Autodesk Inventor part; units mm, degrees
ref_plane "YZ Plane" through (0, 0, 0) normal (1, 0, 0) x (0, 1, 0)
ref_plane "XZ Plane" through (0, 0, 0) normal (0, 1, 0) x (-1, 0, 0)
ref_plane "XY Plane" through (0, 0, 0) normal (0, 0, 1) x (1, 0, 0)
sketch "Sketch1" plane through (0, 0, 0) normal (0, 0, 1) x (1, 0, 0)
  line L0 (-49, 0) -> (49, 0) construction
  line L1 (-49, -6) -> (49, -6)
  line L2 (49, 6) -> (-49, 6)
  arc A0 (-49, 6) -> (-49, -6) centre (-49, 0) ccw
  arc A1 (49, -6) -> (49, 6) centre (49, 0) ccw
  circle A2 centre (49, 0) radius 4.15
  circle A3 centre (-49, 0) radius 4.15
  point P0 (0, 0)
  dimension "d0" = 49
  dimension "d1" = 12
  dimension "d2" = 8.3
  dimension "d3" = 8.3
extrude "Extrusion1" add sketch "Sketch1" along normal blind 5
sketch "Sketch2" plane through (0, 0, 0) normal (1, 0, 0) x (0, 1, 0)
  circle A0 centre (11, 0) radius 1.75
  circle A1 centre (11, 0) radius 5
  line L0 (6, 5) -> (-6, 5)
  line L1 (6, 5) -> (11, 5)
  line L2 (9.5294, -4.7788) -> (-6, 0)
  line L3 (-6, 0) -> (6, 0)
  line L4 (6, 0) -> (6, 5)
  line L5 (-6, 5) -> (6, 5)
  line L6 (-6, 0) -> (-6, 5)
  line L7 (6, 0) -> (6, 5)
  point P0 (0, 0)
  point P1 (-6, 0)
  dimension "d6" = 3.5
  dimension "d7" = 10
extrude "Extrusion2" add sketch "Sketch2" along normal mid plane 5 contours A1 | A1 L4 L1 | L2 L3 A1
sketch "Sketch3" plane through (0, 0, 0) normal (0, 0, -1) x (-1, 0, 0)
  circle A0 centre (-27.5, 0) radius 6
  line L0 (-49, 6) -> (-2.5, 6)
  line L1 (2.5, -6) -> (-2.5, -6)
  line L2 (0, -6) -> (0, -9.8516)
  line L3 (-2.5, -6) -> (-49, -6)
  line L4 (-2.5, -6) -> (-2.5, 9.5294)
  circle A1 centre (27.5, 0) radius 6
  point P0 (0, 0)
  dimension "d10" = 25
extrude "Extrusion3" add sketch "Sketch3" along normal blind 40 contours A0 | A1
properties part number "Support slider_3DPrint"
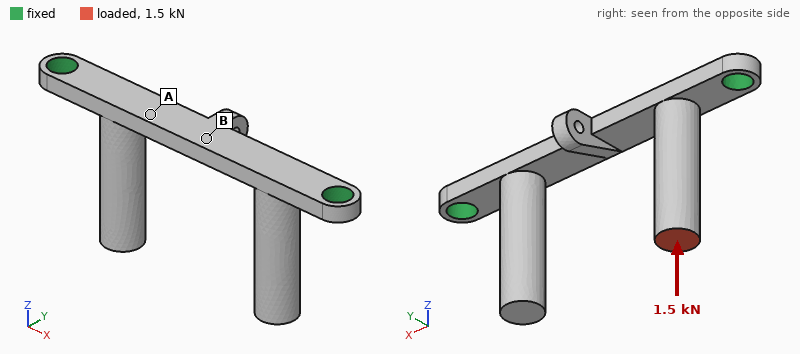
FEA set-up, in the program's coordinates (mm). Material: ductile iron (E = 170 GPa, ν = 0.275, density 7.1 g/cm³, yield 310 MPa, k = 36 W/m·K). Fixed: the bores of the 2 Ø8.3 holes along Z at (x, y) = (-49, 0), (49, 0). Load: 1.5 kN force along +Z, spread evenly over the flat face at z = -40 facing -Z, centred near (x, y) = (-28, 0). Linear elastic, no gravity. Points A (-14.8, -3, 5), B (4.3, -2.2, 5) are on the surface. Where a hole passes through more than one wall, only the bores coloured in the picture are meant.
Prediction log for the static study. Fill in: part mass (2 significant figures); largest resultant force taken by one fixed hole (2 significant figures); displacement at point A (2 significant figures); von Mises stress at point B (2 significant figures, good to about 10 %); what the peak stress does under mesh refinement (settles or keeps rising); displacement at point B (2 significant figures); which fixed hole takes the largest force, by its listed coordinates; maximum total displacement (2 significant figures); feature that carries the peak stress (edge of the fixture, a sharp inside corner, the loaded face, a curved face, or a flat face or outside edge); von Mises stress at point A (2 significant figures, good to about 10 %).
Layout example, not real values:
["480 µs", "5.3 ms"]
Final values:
["110 g", "1.3 kN", "0.11 mm", "42 MPa", "keeps rising", "0.093 mm", "(-49, 0)", "0.21 mm", "edge of the fixture", "110 MPa"]
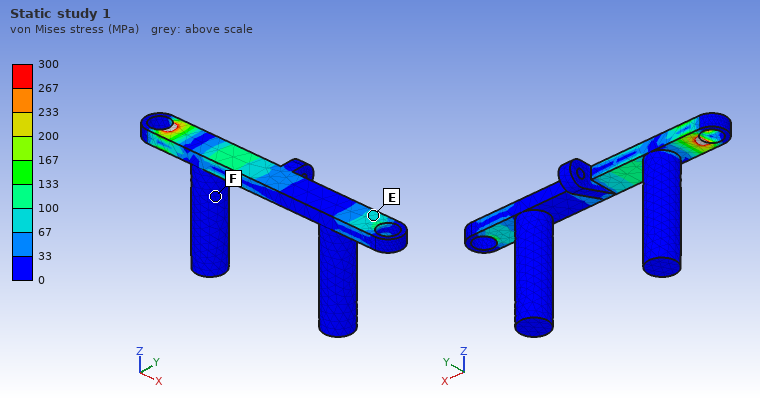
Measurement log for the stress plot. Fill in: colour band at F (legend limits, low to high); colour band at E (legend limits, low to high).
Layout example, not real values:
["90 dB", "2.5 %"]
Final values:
["0 to 33 MPa", "67 to 100 MPa"]
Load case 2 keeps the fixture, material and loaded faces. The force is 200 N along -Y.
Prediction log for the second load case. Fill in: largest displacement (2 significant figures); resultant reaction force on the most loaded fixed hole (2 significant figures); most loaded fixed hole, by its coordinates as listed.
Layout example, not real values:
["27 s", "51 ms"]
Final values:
["0.19 mm", "180 N", "(-49, 0)"]
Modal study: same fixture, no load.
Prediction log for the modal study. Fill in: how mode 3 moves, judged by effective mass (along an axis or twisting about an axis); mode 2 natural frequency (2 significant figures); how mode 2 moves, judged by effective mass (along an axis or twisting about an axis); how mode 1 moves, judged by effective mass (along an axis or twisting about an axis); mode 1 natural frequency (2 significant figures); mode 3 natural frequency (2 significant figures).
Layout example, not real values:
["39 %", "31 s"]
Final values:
["twisting about Z", "1400 Hz", "along Y", "along Z", "1300 Hz", "1800 Hz"]
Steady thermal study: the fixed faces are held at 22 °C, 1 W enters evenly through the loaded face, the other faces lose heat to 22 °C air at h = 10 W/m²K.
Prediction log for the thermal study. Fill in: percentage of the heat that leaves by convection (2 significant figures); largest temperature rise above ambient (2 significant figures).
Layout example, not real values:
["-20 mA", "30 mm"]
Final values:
["23 %", "14 K"]
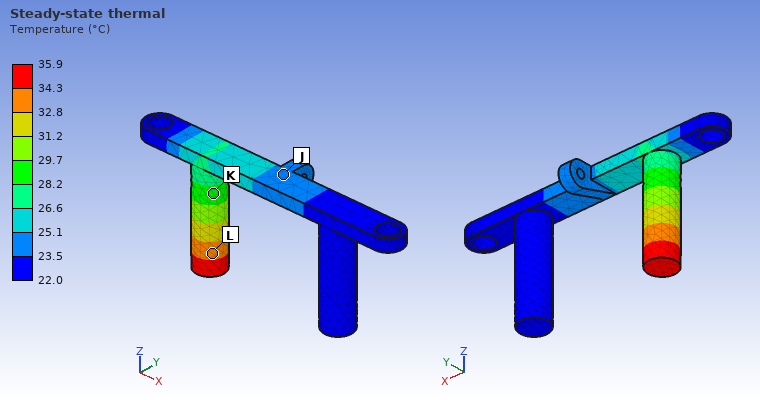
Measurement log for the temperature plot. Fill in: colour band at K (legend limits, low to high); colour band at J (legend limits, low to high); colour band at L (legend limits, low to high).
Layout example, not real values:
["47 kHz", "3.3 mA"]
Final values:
["28.2 to 29.7 °C", "23.5 to 25.1 °C", "32.8 to 34.3 °C"]
